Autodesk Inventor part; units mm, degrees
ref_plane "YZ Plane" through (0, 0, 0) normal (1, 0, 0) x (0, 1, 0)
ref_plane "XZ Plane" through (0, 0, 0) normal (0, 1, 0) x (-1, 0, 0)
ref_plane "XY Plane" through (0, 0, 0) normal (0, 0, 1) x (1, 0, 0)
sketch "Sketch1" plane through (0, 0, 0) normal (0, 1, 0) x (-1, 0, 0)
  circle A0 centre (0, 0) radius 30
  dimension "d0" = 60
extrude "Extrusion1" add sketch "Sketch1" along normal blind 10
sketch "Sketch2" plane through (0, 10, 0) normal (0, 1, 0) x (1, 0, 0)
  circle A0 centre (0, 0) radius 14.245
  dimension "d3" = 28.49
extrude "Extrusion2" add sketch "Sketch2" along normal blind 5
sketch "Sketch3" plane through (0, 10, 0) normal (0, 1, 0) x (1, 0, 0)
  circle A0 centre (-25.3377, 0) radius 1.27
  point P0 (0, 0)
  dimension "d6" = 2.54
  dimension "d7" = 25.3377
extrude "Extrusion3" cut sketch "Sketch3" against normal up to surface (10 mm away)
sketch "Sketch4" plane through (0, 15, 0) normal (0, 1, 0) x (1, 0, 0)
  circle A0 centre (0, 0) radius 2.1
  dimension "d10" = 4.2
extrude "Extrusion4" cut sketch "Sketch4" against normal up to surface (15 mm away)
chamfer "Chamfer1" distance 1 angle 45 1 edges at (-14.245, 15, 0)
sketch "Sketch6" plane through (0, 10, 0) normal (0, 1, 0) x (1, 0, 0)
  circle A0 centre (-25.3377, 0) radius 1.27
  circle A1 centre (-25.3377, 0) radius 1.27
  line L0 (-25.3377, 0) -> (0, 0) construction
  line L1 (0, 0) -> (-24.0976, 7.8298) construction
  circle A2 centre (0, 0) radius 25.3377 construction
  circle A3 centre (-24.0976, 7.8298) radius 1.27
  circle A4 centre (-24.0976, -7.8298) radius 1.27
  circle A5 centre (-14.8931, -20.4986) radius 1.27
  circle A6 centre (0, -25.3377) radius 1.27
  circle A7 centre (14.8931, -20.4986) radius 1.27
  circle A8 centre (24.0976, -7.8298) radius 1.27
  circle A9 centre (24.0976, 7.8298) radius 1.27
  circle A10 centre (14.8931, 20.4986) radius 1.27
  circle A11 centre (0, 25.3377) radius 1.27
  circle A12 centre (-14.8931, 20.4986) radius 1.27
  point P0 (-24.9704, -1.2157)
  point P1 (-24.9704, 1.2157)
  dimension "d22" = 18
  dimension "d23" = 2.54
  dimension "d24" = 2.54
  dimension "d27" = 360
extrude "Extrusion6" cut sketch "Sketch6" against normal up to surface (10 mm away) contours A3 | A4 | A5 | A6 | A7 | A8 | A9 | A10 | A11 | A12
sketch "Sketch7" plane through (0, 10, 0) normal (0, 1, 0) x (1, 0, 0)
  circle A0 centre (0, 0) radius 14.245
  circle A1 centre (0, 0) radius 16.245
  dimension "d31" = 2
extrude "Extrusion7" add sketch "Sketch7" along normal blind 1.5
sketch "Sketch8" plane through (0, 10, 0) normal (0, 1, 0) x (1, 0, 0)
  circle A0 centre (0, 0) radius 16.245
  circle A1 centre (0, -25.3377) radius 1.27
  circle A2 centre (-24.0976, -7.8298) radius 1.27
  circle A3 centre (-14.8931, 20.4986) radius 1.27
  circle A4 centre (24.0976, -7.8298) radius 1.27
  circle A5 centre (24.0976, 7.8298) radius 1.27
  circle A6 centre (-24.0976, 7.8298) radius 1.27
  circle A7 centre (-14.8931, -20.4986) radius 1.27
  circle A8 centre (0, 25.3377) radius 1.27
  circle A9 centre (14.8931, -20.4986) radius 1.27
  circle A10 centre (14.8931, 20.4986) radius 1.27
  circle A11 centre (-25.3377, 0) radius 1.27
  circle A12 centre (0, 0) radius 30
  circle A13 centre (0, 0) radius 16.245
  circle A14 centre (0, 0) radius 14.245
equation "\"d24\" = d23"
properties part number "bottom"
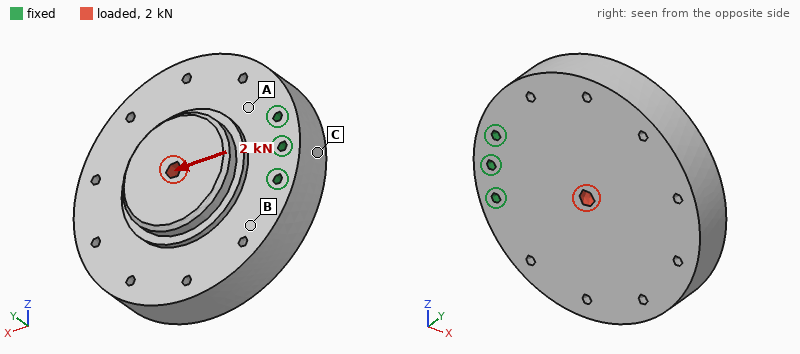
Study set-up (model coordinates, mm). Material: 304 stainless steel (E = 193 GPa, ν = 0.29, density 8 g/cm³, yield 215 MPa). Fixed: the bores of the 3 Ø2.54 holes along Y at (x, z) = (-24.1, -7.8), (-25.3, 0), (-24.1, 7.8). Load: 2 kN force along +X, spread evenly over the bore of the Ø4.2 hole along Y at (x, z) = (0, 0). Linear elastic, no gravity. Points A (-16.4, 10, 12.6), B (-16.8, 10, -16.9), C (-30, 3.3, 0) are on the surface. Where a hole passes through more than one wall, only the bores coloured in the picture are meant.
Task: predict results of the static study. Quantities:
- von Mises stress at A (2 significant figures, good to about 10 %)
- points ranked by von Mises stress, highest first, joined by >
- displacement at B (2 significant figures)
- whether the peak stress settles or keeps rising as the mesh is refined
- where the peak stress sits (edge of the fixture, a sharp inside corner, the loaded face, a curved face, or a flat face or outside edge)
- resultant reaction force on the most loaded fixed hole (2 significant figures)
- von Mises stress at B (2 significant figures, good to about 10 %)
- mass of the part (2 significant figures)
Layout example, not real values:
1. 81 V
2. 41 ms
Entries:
1. 9.3 MPa
2. A > B > C
3. 1.0 µm
4. keeps rising
5. edge of the fixture
6. 760 N
7. 5.4 MPa
8. 250 g
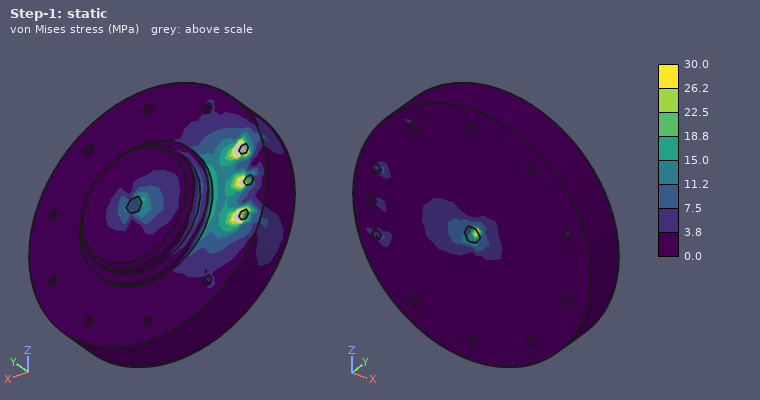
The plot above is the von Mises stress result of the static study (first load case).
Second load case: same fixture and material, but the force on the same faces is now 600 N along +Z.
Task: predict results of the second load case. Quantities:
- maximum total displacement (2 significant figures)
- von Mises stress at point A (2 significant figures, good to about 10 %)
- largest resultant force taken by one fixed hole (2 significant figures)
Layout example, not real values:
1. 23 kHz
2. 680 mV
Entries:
1. 3.6 µm
2. 3.9 MPa
3. 860 N
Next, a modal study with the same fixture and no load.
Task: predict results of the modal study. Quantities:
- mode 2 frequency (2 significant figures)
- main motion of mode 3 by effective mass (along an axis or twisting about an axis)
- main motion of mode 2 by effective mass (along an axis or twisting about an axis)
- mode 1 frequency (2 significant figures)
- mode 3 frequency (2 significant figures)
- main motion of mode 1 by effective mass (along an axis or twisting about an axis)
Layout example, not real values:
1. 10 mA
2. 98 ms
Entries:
1. 4700 Hz
2. twisting about X
3. along Z
4. 2500 Hz
5. 5800 Hz
6. along Y
